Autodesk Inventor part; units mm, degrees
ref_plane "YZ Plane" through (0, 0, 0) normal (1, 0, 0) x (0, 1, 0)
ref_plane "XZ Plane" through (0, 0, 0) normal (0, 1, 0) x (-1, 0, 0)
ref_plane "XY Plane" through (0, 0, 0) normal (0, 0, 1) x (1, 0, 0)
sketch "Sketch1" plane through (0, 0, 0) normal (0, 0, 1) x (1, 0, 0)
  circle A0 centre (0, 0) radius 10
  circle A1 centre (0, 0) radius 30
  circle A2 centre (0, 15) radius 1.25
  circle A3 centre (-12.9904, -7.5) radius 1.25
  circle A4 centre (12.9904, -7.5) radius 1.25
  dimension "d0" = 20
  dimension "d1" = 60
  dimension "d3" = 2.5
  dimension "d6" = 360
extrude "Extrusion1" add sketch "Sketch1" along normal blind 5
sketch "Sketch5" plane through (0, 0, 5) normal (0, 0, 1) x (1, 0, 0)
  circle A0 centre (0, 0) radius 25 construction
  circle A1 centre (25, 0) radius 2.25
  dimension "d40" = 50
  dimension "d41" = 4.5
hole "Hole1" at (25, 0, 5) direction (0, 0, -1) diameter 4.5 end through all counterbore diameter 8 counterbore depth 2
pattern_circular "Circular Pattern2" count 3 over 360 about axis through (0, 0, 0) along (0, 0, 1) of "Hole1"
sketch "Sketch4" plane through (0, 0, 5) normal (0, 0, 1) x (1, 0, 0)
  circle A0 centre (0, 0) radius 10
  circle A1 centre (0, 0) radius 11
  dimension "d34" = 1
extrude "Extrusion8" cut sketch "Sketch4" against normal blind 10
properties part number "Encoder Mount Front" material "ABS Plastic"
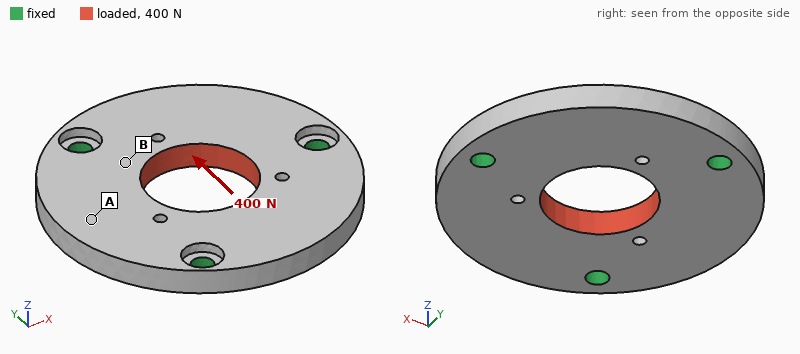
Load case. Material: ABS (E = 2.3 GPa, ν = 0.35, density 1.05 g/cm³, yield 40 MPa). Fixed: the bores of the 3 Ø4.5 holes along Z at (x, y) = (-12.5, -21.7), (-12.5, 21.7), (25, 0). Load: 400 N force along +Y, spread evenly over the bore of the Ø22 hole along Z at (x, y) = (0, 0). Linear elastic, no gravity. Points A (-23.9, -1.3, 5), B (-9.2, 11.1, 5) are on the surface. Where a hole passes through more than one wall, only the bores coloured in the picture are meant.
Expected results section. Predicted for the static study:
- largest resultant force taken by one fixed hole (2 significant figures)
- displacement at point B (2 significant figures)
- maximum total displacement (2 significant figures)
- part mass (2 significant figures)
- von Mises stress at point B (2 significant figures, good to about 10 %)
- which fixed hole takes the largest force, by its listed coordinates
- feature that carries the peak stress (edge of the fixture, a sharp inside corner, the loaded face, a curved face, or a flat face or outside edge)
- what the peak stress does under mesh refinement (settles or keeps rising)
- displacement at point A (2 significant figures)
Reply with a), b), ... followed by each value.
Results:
a) 140 N
b) 13 µm
c) 33 µm
d) 12 g
e) 1.9 MPa
f) (25, 0)
g) edge of the fixture
h) keeps rising
i) 7.1 µm
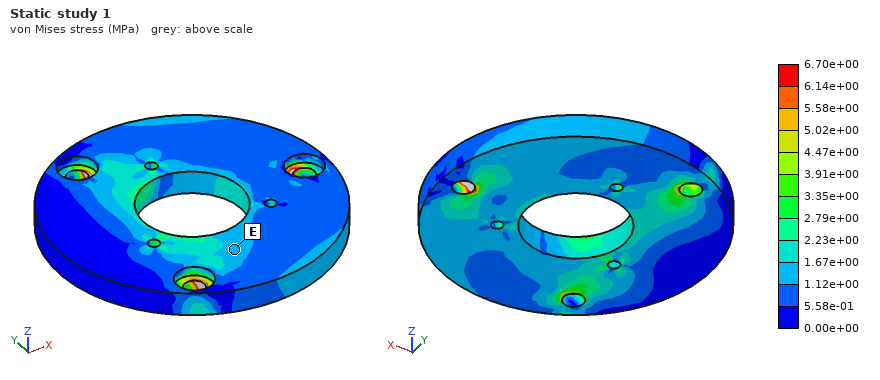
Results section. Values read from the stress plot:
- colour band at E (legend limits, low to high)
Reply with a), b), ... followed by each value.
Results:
a) 1.12e+00 to 1.67e+00 MPa
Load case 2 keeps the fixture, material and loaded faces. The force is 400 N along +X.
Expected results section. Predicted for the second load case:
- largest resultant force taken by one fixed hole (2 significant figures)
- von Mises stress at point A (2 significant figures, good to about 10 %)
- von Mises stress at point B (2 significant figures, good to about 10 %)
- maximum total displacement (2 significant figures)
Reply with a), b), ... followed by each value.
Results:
a) 140 N
b) 1.1 MPa
c) 1.2 MPa
d) 37 µm
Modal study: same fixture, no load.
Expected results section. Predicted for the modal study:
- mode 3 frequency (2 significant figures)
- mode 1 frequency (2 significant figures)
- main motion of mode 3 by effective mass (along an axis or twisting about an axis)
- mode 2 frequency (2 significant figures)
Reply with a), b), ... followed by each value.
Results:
a) 2600 Hz
b) 2100 Hz
c) along Z
d) 2100 Hz
